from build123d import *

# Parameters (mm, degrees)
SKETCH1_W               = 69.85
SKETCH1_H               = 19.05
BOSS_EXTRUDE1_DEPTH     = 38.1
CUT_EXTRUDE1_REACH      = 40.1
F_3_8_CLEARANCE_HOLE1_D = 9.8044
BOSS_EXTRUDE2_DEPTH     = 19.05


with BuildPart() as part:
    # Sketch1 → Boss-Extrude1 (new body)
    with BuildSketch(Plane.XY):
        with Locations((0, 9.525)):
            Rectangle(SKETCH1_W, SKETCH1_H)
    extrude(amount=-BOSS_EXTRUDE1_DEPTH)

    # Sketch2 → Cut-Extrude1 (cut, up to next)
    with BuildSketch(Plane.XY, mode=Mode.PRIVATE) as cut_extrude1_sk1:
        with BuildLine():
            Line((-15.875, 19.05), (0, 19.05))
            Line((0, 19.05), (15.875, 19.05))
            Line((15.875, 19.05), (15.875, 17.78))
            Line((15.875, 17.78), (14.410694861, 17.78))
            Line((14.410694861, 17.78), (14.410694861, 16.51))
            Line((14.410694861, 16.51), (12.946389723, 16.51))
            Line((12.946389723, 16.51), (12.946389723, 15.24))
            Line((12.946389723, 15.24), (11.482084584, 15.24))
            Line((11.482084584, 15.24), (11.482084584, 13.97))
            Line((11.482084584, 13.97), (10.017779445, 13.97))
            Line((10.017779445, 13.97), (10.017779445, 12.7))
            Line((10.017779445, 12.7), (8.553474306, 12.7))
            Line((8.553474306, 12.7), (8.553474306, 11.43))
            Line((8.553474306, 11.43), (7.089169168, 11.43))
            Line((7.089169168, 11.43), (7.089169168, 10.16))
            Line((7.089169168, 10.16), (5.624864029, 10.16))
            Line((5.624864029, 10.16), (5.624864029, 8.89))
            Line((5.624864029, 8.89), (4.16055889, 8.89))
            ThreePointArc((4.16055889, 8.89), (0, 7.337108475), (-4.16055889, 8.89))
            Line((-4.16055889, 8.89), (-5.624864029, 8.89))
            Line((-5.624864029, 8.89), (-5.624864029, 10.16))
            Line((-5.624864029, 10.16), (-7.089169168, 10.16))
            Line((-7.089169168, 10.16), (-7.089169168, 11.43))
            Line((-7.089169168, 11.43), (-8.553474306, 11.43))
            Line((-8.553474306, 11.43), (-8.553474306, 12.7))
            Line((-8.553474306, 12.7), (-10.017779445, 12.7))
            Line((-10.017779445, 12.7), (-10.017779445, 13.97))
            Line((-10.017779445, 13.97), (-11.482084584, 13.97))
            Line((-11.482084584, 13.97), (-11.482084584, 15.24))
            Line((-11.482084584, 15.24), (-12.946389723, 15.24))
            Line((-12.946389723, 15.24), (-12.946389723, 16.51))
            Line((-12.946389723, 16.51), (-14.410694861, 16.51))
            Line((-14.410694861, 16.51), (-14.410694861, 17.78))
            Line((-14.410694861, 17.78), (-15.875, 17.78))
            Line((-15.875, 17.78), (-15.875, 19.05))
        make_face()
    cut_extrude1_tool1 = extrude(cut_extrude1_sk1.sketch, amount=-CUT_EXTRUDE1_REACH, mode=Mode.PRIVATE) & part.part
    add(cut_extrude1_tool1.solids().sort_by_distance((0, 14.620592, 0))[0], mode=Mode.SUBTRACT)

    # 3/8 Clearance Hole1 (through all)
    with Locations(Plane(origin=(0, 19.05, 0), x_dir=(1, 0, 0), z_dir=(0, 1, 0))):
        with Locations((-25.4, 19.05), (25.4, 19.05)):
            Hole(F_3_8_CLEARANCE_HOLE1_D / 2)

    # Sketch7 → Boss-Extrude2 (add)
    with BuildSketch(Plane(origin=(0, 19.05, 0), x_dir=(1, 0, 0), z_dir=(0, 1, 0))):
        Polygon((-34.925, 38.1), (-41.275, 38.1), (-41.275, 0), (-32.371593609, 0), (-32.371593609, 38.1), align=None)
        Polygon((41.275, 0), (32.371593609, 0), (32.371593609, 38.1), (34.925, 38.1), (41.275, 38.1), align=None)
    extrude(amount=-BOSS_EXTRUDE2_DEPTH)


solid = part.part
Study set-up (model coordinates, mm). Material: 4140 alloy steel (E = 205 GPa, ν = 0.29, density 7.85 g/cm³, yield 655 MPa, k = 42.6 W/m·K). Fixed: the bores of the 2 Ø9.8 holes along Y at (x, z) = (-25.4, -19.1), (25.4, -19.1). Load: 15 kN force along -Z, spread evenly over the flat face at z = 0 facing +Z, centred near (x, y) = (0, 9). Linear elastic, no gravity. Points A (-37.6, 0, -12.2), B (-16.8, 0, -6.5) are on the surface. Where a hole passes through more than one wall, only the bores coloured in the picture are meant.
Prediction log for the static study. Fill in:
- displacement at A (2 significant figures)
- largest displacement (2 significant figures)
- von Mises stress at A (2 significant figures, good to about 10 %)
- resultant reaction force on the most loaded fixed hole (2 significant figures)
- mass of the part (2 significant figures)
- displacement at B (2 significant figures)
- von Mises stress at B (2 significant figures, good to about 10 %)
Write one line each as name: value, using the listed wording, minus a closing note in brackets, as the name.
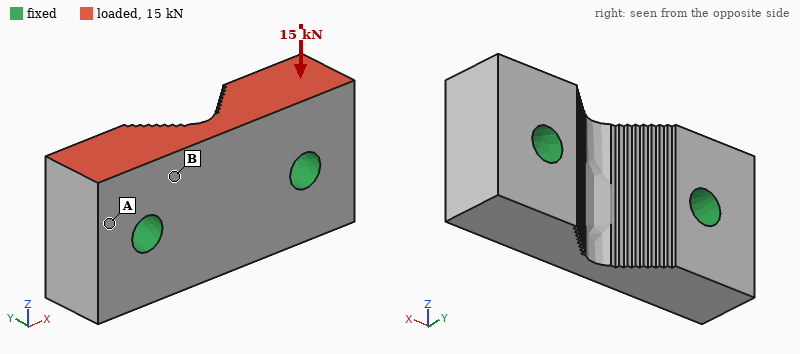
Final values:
displacement at A: 0.78 µm
largest displacement: 2.3 µm
von Mises stress at A: 7.8 MPa
resultant reaction force on the most loaded fixed hole: 7.5 kN
mass of the part: 380 g
displacement at B: 1.1 µm
von Mises stress at B: 13 MPa
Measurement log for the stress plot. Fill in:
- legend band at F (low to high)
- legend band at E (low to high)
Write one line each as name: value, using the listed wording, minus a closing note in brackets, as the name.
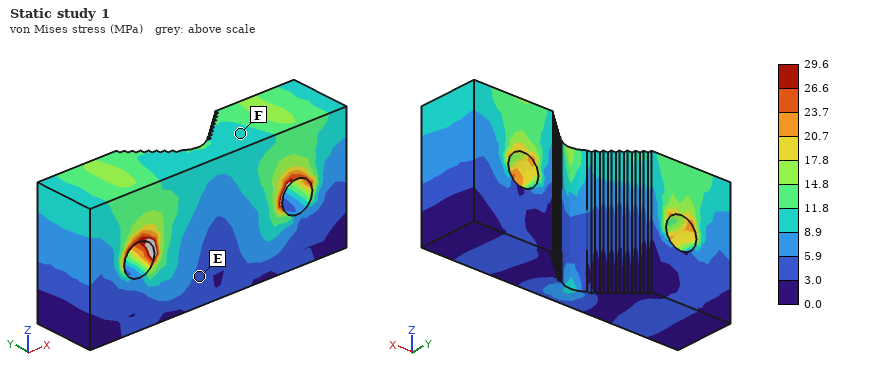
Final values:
legend band at F: 8.9 to 11.8 MPa
legend band at E: 3.0 to 5.9 MPa
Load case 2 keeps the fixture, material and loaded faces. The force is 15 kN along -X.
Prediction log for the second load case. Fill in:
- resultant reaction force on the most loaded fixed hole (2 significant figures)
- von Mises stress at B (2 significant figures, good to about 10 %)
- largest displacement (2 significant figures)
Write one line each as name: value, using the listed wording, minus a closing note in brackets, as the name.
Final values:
resultant reaction force on the most loaded fixed hole: 8.3 kN
von Mises stress at B: 28 MPa
largest displacement: 6.8 µm
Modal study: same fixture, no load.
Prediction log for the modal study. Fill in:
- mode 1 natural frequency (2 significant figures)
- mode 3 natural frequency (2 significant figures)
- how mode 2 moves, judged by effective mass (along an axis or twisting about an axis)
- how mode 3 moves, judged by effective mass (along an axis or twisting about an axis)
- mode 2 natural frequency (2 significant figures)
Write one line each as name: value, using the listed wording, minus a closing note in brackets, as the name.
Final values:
mode 1 natural frequency: 22 kHz
mode 3 natural frequency: 26 kHz
how mode 2 moves, judged by effective mass: along Y
how mode 3 moves, judged by effective mass: twisting about X
mode 2 natural frequency: 25 kHz
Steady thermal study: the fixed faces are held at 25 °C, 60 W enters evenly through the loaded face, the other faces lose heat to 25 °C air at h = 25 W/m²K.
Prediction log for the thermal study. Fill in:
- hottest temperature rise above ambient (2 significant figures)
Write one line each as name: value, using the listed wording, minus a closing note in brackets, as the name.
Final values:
hottest temperature rise above ambient: 22 K
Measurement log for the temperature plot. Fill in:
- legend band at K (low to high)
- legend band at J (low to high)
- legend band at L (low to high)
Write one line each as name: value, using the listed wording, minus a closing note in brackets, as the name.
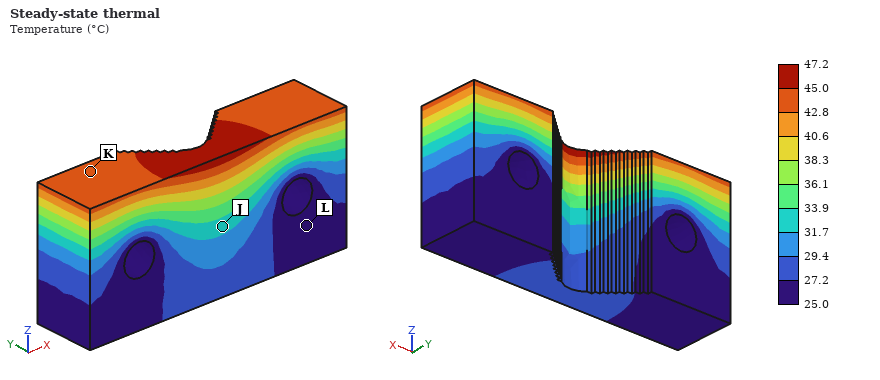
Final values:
legend band at K: 42.8 to 45.0 °C
legend band at J: 31.7 to 33.9 °C
legend band at L: 25.0 to 27.2 °C
